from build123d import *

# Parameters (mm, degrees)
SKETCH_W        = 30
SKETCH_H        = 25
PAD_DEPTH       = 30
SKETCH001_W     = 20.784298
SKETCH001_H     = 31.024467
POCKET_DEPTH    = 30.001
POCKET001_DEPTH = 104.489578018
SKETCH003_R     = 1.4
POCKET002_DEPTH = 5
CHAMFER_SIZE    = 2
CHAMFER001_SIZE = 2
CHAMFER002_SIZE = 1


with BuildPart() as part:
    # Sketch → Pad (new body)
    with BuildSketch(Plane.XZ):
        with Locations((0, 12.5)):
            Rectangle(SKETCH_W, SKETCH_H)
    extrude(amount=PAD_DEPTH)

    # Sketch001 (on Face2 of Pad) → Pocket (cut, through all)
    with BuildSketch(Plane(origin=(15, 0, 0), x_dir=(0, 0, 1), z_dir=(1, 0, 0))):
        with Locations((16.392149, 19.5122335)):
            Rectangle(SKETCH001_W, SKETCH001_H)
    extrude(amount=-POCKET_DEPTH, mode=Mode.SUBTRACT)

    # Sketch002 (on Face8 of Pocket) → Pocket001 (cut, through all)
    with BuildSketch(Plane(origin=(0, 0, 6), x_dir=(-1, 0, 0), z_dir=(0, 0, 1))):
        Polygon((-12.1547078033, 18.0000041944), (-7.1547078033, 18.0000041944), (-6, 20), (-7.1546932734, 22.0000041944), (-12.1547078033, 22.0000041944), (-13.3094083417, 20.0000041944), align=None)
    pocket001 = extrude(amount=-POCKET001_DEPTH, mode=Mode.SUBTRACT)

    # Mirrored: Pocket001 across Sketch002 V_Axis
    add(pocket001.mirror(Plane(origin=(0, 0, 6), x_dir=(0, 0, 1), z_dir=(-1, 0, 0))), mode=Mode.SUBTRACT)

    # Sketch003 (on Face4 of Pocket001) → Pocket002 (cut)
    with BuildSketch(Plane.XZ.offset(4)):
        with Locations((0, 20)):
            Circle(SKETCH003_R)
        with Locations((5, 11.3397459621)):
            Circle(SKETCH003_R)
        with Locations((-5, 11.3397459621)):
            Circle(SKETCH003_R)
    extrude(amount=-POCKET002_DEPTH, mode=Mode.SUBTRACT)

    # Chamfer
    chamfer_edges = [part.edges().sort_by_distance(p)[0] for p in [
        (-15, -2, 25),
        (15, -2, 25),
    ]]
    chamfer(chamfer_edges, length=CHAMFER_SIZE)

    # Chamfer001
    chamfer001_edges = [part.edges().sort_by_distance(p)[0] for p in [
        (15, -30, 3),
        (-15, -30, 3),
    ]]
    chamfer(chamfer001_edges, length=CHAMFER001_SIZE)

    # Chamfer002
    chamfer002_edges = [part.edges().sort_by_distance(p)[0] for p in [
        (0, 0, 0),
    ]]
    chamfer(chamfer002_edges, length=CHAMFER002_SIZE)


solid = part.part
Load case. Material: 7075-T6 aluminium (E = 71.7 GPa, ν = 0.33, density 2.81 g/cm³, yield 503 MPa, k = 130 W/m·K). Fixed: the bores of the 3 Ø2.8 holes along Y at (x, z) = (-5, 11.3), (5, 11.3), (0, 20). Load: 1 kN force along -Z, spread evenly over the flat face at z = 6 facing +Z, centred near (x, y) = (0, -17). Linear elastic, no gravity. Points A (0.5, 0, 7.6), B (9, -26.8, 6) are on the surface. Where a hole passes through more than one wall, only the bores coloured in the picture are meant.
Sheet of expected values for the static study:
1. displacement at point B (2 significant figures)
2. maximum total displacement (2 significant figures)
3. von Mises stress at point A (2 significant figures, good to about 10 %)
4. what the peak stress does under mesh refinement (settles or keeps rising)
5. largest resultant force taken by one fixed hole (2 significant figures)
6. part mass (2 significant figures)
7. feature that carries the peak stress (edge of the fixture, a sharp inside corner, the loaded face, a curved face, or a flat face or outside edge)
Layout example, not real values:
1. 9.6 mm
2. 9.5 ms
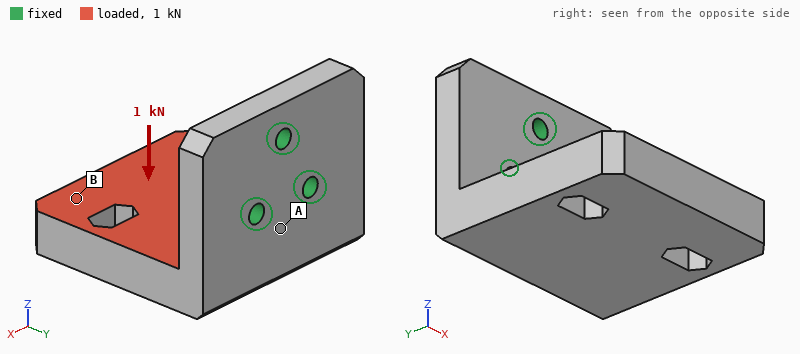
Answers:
1. 0.29 mm
2. 0.34 mm
3. 160 MPa
4. keeps rising
5. 500 N
6. 20 g
7. edge of the fixture
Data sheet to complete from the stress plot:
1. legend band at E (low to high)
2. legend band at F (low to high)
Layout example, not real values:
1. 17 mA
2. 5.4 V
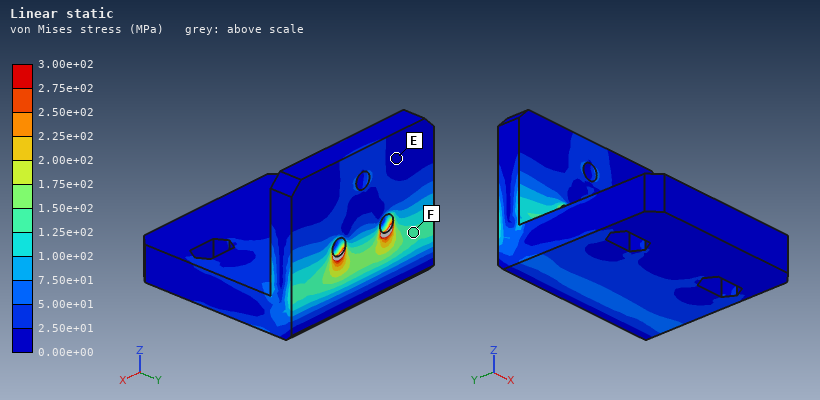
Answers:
1. 0.00e+00 to 2.50e+01 MPa
2. 1.25e+02 to 1.50e+02 MPa
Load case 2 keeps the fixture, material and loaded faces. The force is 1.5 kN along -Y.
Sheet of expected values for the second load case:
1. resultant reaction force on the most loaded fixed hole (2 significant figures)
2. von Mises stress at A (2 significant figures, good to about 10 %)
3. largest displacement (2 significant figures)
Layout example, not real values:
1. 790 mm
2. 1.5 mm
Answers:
1. 840 N
2. 25 MPa
3. 34 µm
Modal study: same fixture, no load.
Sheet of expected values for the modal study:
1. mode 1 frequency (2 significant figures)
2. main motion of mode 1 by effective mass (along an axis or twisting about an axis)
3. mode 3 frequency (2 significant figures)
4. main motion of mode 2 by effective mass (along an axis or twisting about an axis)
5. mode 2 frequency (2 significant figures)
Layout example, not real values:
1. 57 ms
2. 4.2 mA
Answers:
1. 2900 Hz
2. along Z
3. 11 kHz
4. along X
5. 5600 Hz
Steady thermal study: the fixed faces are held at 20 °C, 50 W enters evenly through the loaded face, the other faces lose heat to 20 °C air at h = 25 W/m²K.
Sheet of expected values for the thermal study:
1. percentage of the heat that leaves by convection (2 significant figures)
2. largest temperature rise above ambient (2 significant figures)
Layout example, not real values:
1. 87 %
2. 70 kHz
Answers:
1. 4.3 %
2. 59 K
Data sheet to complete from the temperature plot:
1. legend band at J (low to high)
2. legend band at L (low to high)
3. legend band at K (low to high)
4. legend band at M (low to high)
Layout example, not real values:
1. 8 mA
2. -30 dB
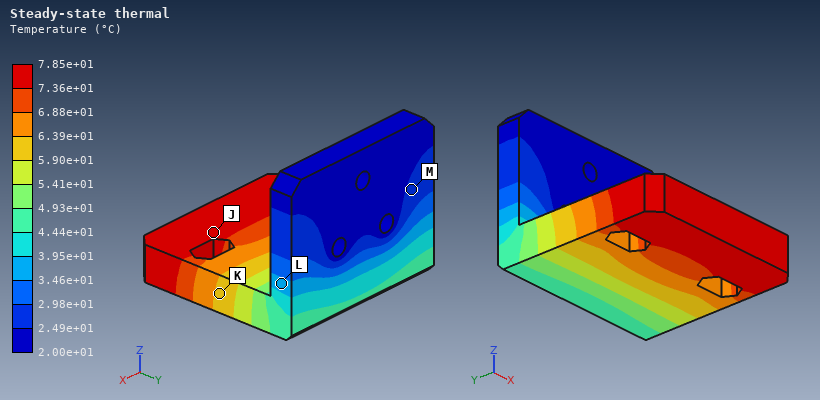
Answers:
1. 7.36e+01 to 7.85e+01 °C
2. 3.46e+01 to 3.95e+01 °C
3. 5.90e+01 to 6.39e+01 °C
4. 2.49e+01 to 2.98e+01 °C
